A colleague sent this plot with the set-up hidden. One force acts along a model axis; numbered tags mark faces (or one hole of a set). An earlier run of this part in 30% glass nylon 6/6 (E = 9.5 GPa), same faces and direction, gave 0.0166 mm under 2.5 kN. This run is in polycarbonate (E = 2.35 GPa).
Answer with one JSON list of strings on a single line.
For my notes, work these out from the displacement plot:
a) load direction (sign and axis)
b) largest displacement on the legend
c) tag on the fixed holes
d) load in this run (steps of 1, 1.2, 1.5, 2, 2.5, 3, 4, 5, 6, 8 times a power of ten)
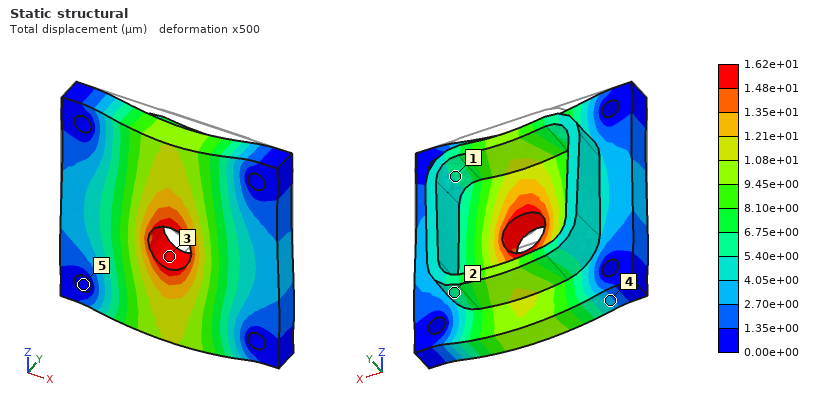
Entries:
["-Z", "1.62e+01 µm", "5", "600 N"]
